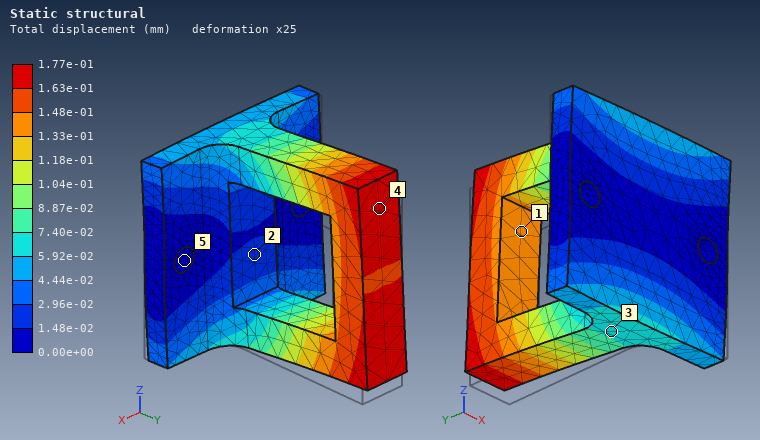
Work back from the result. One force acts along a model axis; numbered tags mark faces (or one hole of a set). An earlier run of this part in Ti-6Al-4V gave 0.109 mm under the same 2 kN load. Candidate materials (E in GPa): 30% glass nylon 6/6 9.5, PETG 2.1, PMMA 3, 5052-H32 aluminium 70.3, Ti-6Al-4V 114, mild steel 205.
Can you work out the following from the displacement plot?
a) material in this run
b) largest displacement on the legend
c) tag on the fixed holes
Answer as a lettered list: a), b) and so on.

a) 5052-H32 aluminium
b) 1.77e-01 mm
c) 5
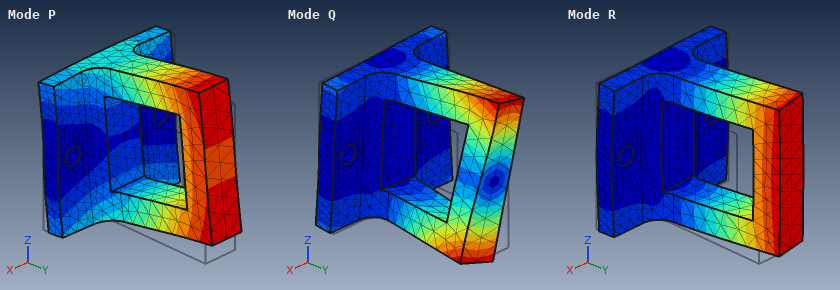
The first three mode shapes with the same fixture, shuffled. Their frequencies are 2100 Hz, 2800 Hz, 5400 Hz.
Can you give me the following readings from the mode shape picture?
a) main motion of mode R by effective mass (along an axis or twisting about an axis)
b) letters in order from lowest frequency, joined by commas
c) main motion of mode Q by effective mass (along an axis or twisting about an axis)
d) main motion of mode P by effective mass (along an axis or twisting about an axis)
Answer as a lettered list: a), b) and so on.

a) along X
b) P, R, Q
c) twisting about Y
d) along Z
